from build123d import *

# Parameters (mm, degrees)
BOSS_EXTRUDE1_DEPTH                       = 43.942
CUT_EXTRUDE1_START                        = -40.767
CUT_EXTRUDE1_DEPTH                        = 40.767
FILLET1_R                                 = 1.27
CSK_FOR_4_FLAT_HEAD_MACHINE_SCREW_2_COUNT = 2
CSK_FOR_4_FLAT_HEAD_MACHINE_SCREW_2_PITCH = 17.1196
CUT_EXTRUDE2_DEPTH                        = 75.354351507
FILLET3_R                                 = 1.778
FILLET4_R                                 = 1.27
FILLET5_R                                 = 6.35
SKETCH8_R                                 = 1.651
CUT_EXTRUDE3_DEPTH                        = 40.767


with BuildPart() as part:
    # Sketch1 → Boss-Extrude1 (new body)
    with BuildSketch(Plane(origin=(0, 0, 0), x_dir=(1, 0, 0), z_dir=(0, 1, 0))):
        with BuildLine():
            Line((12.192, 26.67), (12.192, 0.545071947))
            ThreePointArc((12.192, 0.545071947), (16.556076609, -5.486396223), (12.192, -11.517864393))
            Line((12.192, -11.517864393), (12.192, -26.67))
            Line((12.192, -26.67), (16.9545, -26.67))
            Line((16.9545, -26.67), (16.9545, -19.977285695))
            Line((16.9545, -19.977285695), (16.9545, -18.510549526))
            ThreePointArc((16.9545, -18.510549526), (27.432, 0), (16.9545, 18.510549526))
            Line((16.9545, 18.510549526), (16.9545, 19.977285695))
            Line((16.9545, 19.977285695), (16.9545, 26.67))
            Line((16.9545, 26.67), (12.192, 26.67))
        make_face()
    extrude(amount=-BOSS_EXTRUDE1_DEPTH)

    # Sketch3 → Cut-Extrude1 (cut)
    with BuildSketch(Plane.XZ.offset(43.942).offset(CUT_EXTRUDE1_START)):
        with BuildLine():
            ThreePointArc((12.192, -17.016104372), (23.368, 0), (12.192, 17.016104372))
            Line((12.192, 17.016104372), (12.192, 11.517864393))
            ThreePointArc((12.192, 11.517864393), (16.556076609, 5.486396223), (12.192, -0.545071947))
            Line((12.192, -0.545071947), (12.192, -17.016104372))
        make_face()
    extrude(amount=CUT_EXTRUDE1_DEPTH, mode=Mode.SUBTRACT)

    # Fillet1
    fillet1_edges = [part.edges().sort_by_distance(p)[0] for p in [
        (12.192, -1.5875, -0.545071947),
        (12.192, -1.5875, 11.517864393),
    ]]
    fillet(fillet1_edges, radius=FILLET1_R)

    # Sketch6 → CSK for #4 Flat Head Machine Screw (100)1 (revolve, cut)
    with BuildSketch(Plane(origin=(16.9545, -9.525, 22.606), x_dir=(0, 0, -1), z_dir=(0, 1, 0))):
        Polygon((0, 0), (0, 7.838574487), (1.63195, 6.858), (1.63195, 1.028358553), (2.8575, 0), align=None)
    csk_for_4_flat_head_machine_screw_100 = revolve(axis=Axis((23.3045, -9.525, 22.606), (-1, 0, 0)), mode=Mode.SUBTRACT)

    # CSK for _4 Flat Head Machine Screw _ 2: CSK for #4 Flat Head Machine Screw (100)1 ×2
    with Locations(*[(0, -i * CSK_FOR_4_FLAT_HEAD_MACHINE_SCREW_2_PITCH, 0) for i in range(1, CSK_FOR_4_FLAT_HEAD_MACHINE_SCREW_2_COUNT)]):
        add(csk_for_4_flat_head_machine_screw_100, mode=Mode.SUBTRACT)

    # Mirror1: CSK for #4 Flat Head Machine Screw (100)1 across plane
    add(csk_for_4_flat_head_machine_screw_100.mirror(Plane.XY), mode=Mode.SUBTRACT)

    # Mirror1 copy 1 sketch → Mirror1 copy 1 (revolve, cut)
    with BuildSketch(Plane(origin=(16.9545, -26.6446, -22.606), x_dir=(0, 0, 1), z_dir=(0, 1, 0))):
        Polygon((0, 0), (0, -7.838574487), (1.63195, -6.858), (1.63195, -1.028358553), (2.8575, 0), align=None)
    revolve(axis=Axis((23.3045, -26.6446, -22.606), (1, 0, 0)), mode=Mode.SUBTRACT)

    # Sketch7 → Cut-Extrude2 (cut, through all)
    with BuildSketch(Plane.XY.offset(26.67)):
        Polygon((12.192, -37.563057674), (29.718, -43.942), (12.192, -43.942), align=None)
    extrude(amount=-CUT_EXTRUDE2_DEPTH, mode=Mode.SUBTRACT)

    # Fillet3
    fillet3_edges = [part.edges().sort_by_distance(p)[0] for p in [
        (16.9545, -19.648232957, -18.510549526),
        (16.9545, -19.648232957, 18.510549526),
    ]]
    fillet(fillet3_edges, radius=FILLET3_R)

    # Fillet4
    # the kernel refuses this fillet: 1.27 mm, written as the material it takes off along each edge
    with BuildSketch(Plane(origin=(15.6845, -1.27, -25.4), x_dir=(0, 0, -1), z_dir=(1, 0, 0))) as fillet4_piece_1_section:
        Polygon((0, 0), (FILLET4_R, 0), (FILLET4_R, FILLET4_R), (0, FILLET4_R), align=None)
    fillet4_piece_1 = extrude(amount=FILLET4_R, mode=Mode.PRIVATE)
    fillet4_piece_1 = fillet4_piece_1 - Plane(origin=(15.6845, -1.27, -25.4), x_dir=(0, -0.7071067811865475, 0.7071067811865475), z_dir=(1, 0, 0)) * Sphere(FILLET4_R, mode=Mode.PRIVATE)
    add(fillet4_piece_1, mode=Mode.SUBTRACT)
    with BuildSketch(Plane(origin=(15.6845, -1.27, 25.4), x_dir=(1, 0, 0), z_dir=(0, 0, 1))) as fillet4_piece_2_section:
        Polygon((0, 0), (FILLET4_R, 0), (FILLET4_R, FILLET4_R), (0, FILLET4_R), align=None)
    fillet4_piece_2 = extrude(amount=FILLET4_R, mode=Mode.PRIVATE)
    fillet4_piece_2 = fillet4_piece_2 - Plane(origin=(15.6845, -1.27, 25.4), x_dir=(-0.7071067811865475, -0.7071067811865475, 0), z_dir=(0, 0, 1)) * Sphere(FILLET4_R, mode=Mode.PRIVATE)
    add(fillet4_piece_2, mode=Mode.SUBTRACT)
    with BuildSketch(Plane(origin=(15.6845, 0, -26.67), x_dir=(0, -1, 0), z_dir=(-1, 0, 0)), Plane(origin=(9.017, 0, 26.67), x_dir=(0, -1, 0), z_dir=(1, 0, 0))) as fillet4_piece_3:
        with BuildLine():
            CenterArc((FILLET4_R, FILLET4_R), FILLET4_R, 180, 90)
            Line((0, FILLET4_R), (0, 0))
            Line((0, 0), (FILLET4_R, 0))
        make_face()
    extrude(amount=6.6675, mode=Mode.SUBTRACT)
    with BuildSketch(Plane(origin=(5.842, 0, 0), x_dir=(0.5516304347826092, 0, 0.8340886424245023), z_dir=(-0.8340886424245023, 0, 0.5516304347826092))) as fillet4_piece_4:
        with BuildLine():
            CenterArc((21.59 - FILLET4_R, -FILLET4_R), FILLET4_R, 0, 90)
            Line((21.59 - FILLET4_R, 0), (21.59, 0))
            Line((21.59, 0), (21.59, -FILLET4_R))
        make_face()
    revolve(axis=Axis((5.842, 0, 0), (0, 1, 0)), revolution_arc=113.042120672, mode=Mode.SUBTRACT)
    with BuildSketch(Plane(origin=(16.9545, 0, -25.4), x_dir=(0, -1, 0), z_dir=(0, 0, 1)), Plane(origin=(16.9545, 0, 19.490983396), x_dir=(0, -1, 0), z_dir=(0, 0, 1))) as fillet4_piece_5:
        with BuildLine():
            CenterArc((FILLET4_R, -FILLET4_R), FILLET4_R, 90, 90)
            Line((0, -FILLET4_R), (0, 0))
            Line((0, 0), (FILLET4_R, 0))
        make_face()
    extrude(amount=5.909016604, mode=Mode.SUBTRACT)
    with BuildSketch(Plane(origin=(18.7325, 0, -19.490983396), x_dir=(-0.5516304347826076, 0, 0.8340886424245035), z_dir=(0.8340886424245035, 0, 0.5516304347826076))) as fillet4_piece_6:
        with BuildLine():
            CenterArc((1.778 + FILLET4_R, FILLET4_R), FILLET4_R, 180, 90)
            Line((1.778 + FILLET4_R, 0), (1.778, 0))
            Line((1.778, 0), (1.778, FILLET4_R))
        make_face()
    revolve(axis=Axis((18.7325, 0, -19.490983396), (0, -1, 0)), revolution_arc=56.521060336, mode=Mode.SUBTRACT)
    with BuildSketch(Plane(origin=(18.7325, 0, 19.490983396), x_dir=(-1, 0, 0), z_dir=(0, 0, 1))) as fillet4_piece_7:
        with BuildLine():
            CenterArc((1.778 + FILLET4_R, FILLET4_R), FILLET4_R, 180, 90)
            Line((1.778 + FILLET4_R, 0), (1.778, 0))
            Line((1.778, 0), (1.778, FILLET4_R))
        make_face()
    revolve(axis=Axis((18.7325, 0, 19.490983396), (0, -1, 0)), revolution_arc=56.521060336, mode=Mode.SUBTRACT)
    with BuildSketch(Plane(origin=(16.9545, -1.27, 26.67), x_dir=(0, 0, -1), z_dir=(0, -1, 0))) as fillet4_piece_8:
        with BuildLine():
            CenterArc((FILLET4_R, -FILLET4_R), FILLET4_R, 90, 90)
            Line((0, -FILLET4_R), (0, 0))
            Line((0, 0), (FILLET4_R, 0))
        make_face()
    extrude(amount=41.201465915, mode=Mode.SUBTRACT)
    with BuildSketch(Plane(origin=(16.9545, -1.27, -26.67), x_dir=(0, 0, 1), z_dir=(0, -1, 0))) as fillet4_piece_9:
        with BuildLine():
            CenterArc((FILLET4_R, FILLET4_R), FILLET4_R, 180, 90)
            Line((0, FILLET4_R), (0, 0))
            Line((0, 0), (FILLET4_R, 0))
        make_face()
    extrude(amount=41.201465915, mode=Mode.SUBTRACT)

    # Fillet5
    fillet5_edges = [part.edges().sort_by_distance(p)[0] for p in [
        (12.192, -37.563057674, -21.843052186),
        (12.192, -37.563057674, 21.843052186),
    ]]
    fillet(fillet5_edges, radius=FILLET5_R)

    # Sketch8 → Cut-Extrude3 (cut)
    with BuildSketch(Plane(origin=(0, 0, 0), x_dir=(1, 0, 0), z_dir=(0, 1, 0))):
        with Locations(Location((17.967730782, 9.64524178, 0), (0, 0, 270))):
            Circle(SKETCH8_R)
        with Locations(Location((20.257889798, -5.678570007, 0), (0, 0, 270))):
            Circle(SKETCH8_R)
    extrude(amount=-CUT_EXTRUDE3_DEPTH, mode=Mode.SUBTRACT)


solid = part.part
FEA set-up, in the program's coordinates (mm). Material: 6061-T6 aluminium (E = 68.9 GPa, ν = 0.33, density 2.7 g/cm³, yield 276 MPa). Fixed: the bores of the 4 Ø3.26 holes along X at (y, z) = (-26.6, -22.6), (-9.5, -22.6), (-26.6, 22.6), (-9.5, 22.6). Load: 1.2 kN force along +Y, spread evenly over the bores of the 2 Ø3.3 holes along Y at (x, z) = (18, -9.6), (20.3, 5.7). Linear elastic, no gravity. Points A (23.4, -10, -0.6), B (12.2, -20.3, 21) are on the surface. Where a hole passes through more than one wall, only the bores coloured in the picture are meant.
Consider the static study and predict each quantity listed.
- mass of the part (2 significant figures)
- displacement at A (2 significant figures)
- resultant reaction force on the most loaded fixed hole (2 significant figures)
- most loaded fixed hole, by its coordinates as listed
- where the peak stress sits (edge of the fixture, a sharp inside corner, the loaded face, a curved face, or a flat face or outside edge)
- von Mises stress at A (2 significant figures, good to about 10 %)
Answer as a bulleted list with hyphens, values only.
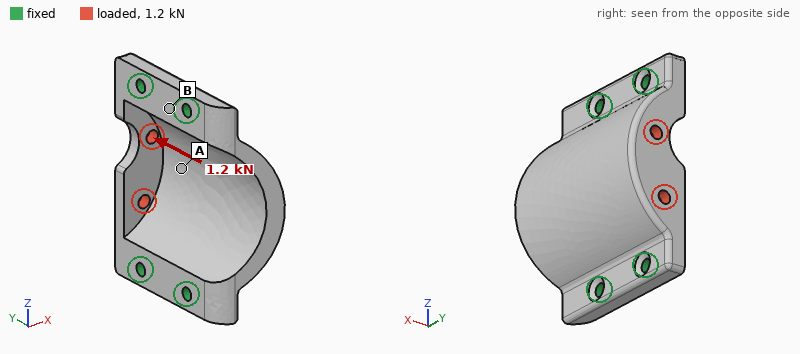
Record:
- 29 g
- 6.3 µm
- 440 N
- (-9.5, -22.6)
- the loaded face
- 15 MPa
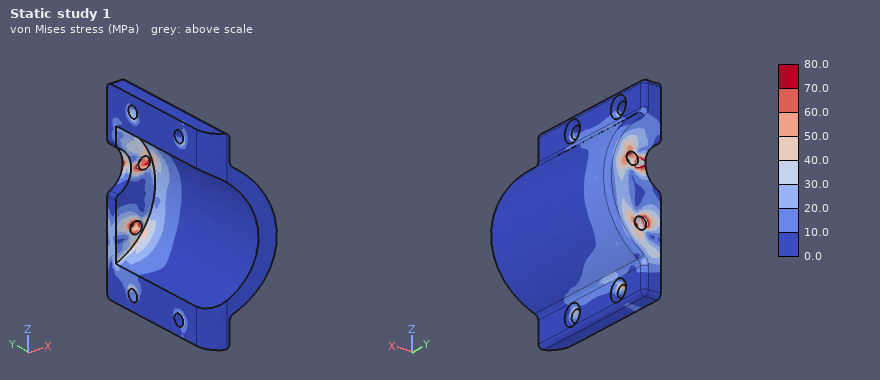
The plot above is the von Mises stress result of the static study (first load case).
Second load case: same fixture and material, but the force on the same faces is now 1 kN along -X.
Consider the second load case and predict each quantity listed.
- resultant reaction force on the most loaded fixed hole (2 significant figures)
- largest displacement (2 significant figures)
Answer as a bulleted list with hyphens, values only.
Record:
- 980 N
- 26 µm
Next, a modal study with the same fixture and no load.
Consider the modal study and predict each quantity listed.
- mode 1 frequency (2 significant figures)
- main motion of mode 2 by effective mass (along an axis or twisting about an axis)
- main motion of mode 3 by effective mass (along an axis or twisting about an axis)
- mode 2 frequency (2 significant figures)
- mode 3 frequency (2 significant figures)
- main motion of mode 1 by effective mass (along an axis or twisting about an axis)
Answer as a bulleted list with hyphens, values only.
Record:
- 12 kHz
- along Z
- along X
- 16 kHz
- 18 kHz
- along Y
